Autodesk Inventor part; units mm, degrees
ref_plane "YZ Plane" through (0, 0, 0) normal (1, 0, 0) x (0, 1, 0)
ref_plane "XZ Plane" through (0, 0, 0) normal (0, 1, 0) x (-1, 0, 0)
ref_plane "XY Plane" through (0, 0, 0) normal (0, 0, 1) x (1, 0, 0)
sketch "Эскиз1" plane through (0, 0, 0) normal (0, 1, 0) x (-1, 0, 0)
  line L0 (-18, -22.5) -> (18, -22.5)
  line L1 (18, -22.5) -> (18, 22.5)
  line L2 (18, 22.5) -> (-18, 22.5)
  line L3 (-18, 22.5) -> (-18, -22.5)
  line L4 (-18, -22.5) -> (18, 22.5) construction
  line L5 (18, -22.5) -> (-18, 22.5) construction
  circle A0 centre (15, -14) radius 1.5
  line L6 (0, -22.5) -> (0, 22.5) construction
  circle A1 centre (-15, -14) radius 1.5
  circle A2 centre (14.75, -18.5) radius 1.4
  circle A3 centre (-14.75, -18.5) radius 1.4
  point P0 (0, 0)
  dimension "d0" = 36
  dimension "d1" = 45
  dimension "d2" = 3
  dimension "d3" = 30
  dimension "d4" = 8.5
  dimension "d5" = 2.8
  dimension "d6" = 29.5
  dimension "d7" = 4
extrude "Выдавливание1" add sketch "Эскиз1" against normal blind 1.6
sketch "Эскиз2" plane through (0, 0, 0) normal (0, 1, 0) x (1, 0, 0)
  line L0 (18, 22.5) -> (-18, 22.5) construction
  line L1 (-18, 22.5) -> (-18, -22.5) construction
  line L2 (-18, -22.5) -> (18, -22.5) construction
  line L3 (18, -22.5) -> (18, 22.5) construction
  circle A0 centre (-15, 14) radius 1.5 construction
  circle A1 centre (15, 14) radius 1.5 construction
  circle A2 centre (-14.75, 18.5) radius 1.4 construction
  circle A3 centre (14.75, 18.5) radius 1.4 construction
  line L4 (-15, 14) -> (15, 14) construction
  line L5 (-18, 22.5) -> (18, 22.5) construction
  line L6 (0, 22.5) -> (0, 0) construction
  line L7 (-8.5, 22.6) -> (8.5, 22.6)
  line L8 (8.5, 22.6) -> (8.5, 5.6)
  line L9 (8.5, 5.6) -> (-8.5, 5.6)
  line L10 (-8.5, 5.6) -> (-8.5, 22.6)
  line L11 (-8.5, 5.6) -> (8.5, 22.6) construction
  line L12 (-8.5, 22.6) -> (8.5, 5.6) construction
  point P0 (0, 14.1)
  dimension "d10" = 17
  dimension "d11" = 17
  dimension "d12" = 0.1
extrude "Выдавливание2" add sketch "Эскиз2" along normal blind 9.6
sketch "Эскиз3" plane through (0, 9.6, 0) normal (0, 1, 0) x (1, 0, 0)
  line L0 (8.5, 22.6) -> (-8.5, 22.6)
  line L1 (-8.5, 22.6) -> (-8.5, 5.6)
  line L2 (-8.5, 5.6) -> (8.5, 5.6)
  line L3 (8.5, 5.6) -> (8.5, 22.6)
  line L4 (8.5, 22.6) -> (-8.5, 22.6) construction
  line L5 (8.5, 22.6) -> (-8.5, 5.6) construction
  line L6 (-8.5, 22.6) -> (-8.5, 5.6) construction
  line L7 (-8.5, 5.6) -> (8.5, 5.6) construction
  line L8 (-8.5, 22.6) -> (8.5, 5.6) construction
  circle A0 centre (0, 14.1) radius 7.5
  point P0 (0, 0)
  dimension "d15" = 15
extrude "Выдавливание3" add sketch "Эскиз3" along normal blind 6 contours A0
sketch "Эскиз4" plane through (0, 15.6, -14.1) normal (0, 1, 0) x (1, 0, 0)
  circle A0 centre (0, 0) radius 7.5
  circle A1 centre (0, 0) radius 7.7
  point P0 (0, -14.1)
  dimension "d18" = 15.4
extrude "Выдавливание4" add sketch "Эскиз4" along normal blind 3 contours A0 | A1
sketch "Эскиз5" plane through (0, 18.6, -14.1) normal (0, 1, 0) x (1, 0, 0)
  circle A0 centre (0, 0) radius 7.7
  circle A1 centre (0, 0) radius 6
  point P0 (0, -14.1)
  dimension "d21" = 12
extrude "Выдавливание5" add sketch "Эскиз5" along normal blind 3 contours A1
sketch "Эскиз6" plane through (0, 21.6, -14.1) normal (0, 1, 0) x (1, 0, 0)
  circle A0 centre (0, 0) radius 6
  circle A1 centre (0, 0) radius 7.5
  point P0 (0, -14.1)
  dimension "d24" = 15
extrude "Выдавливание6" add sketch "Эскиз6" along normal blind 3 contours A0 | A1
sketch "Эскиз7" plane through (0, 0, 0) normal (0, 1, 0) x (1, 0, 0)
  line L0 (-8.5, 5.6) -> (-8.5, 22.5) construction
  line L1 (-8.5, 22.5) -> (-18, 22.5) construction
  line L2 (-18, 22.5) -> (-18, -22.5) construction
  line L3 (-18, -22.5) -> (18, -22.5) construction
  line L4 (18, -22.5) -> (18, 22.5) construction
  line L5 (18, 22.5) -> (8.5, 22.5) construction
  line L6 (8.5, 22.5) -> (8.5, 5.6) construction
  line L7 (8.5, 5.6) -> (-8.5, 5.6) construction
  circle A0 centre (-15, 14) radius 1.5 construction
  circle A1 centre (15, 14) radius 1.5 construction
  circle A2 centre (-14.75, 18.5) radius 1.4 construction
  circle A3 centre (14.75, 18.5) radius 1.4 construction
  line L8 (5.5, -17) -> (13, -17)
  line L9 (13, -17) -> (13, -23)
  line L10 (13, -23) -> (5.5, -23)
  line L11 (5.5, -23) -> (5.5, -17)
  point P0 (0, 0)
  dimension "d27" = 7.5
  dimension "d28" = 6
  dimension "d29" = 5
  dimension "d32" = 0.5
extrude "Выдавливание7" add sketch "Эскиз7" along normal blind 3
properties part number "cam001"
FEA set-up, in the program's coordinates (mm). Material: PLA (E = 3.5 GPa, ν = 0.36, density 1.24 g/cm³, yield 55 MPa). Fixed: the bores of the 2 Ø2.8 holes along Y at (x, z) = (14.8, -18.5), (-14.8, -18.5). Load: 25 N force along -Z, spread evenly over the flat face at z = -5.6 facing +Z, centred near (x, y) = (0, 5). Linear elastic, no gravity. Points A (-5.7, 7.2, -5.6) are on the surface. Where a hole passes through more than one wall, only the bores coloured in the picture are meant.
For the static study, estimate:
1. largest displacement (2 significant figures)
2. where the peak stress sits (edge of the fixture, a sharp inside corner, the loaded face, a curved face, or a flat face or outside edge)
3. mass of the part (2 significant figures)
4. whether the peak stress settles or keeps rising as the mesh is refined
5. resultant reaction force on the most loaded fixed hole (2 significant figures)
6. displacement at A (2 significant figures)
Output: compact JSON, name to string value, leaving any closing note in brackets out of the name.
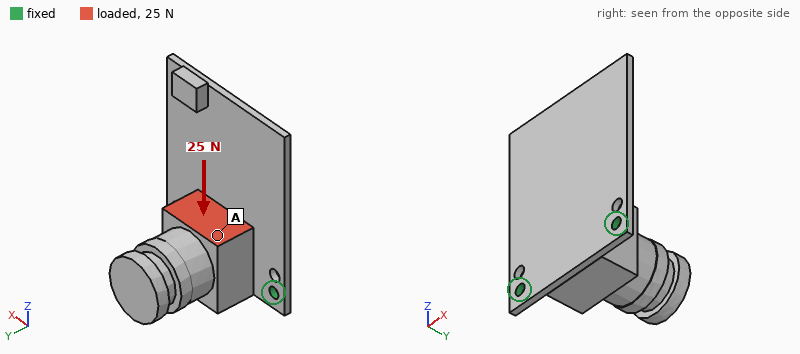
{"largest displacement": "0.66 mm", "where the peak stress sits": "edge of the fixture", "mass of the part": "9.9 g", "whether the peak stress settles or keeps rising as the mesh is refined": "keeps rising", "resultant reaction force on the most loaded fixed hole": "14 N", "displacement at A": "0.23 mm"}
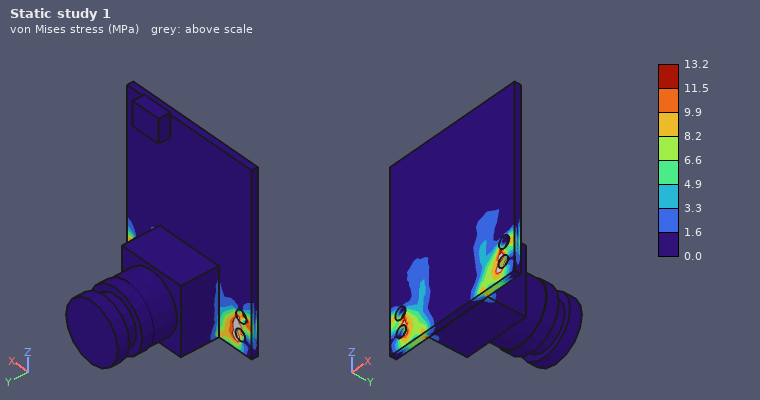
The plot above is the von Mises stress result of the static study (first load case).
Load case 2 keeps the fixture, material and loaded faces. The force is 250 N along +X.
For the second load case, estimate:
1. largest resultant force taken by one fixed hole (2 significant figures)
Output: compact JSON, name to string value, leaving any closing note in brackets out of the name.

{"largest resultant force taken by one fixed hole": "180 N"}
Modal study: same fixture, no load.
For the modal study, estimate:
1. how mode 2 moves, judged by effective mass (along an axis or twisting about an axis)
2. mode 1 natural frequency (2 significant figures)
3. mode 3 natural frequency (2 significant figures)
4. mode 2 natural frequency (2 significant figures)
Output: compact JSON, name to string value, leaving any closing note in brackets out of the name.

{"how mode 2 moves, judged by effective mass": "along Z", "mode 1 natural frequency": "240 Hz", "mode 3 natural frequency": "880 Hz", "mode 2 natural frequency": "720 Hz"}
